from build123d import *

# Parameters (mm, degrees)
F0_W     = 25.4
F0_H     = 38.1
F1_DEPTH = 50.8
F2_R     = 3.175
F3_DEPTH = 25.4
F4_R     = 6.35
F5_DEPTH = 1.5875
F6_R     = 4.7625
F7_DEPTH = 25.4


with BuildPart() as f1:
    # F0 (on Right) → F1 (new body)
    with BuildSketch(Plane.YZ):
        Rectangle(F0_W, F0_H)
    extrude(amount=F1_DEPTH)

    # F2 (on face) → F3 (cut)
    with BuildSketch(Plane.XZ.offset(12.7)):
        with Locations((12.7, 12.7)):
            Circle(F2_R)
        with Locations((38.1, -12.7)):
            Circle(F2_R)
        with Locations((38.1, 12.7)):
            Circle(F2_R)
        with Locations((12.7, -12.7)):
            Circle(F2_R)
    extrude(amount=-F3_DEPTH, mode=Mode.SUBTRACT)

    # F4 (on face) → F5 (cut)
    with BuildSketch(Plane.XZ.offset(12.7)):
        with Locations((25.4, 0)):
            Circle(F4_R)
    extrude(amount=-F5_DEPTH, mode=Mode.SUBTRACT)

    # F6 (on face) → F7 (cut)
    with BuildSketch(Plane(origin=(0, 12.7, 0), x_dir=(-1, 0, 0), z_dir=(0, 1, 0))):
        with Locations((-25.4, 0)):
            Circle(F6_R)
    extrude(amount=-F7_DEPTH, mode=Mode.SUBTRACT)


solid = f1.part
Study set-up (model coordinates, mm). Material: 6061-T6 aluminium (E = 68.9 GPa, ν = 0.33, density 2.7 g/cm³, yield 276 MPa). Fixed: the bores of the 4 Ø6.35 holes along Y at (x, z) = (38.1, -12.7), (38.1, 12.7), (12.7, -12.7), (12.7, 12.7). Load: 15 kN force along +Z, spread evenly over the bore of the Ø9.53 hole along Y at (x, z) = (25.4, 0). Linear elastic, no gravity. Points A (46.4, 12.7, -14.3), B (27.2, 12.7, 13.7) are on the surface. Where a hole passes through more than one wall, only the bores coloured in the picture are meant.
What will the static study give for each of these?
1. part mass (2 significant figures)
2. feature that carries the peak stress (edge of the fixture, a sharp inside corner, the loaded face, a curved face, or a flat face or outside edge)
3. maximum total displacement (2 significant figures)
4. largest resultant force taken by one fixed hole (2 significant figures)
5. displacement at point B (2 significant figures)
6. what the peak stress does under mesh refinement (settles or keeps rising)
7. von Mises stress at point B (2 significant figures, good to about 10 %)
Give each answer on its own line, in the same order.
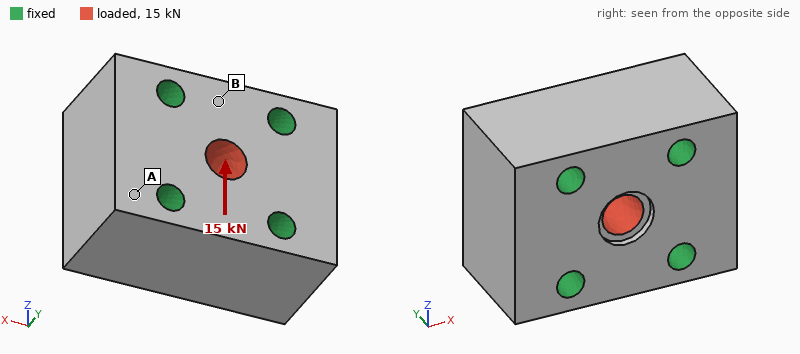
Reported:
120 g
edge of the fixture
4.5 µm
4.1 kN
2.7 µm
keeps rising
6.5 MPa
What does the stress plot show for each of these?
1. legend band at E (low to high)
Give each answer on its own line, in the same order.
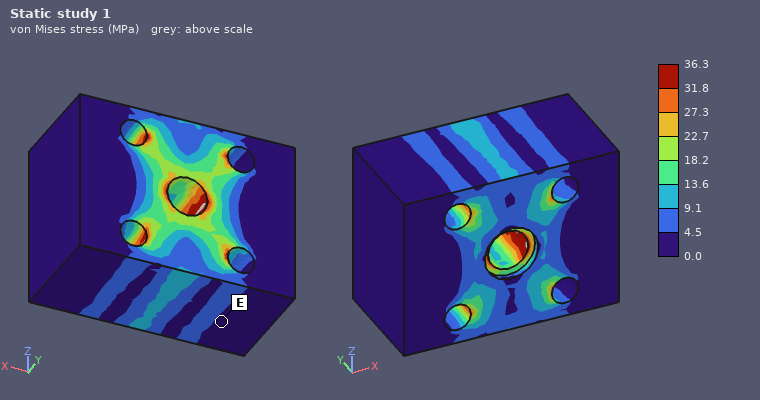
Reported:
0.0 to 4.5 MPa
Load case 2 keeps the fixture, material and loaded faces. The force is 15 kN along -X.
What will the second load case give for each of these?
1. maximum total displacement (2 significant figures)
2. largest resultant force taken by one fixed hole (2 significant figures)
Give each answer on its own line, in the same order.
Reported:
4.1 µm
4.0 kN
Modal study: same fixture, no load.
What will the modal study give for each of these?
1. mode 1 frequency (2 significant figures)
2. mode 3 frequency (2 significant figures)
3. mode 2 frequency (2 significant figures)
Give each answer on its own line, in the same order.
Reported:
49 kHz
57 kHz
49 kHz
